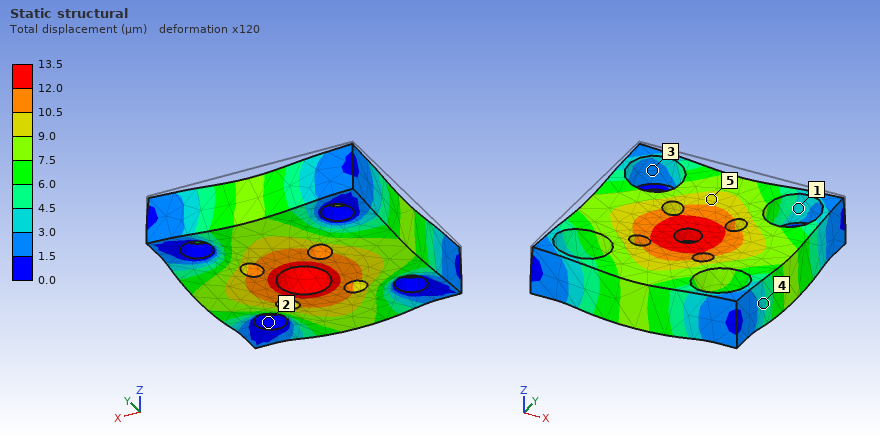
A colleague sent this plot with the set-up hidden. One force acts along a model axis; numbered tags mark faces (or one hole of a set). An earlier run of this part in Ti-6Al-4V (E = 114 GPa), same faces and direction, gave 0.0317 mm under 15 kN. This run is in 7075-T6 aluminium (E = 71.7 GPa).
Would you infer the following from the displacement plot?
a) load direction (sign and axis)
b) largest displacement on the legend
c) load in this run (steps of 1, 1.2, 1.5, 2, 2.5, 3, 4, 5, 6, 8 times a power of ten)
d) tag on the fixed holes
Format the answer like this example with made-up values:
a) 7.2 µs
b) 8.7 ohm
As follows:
a) -Z
b) 13.5 µm
c) 4 kN
d) 2
